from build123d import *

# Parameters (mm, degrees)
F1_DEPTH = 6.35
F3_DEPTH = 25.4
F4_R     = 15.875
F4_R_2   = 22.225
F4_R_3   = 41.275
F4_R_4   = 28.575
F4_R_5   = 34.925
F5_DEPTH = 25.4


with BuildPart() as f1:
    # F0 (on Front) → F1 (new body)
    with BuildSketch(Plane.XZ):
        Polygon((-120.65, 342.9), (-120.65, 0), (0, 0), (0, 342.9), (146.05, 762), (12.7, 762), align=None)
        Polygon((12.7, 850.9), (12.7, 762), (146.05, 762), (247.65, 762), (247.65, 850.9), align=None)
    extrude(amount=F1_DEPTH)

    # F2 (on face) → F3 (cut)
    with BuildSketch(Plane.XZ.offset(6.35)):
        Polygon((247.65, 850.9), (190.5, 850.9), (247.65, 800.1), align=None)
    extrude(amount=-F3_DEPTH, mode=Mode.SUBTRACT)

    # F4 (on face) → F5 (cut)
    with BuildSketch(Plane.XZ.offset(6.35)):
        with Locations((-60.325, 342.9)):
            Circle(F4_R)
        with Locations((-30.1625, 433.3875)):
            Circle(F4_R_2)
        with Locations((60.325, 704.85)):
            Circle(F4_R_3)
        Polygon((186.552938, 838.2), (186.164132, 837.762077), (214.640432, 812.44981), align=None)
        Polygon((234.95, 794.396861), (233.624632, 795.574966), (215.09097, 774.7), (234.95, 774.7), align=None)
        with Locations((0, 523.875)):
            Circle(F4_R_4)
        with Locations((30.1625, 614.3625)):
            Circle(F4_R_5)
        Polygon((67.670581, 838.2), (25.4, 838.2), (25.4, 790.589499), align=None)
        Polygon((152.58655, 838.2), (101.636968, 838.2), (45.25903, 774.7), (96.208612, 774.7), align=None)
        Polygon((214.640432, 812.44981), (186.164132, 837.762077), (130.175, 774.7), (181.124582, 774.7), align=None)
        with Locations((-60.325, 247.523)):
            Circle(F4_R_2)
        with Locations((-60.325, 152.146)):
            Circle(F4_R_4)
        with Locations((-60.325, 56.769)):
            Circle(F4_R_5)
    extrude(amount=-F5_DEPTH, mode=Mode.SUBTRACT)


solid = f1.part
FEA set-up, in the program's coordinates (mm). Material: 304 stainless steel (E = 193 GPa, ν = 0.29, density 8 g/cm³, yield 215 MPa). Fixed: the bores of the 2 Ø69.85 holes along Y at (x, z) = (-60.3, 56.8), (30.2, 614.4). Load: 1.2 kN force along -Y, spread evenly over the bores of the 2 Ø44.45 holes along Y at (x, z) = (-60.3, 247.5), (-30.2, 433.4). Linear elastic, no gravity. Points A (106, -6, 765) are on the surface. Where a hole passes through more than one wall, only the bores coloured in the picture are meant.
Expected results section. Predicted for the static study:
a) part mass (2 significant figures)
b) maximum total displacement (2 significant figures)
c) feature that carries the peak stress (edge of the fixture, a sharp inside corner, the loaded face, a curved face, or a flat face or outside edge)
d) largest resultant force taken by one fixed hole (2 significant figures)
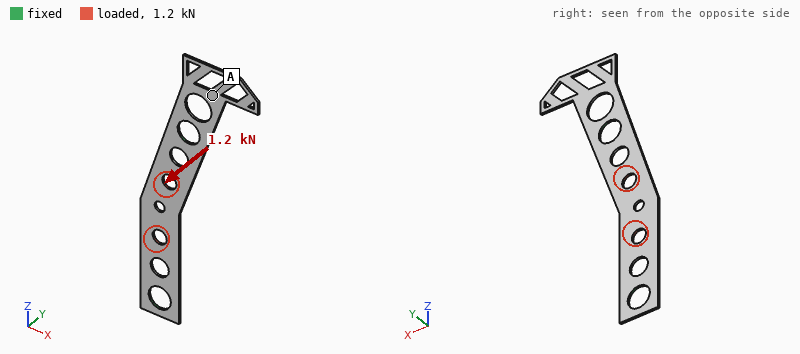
4.3 kg
1.6 mm
a curved face
600 N
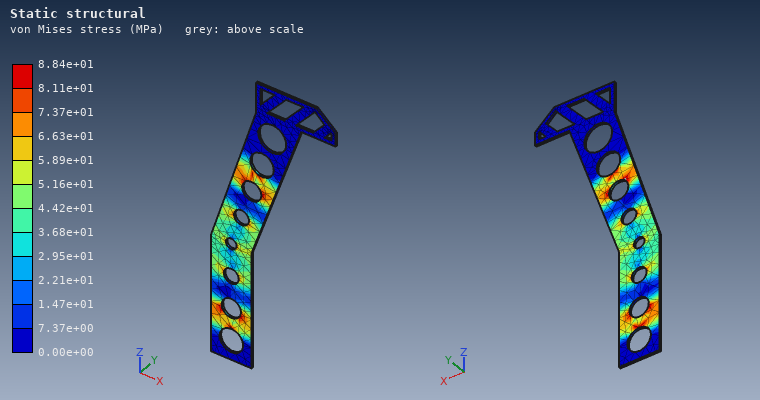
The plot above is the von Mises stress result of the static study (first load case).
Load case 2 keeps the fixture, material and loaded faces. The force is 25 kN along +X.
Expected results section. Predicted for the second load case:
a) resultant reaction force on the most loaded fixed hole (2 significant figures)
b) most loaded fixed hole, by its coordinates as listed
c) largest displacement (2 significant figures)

16 kN
(30.2, 614.4)
0.18 mm
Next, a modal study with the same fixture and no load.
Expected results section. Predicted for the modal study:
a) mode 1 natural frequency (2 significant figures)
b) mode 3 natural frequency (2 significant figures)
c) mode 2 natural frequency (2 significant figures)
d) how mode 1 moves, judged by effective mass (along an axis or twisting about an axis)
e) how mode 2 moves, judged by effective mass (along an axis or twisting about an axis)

67 Hz
170 Hz
120 Hz
along Y
along Y
